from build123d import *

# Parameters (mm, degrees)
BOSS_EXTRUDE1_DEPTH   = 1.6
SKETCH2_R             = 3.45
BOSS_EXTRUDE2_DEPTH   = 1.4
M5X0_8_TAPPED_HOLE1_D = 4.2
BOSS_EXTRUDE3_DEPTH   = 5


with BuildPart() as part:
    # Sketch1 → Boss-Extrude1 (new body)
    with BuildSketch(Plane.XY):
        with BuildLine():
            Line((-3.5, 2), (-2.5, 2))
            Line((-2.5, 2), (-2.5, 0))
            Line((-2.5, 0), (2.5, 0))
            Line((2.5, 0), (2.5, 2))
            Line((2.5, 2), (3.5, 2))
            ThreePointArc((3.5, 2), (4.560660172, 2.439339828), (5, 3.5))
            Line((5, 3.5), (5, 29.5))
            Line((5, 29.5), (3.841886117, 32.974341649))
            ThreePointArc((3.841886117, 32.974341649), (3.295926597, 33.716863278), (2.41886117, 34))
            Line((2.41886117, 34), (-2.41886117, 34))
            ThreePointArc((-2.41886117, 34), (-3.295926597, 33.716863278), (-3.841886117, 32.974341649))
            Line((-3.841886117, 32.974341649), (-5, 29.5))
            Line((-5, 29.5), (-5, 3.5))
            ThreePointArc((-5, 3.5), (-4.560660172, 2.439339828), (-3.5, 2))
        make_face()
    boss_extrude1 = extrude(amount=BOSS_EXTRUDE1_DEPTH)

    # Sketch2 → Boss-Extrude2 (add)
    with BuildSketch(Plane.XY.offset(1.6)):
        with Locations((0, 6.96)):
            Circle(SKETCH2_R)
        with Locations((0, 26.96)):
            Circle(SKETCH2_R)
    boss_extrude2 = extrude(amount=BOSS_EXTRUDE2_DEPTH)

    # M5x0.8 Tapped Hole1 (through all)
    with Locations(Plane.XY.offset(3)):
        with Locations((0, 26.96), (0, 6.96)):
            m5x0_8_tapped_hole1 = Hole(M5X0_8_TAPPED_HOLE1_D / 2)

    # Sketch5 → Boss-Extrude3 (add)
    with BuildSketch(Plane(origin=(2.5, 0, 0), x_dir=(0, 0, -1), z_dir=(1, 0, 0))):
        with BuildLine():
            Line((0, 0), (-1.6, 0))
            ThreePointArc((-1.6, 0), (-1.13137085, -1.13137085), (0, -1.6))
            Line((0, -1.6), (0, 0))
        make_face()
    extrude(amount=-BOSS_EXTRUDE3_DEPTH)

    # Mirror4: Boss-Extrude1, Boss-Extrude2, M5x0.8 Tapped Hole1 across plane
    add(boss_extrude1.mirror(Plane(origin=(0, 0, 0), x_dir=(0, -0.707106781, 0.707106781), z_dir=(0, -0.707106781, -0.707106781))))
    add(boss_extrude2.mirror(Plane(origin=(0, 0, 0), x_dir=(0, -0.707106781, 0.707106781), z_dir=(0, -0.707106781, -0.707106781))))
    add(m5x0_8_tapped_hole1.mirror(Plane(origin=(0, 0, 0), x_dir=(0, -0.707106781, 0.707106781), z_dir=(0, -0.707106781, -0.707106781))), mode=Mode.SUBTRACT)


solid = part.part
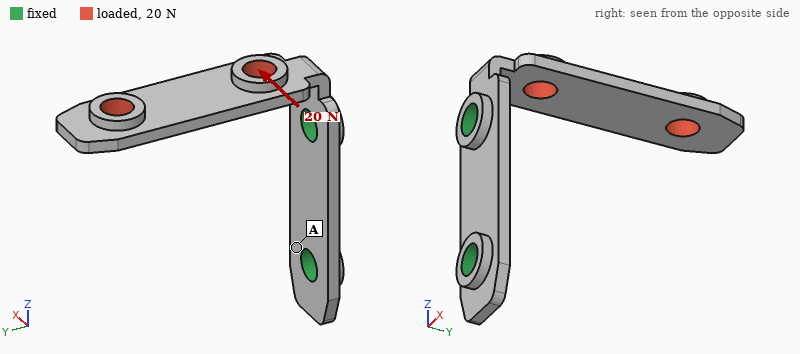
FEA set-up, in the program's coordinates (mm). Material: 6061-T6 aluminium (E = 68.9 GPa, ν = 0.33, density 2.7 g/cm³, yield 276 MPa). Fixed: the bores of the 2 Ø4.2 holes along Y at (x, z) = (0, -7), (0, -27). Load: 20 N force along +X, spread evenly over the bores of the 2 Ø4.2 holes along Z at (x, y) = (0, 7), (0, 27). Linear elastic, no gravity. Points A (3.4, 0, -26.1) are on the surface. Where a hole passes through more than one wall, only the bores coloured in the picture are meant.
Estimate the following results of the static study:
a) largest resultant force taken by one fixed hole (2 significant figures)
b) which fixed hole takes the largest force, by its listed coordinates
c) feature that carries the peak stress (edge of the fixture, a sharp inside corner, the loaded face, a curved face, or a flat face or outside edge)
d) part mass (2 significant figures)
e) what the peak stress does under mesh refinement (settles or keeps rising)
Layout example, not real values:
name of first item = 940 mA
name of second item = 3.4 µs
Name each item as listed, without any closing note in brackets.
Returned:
largest resultant force taken by one fixed hole = 21 N
which fixed hole takes the largest force, by its listed coordinates = (0, -7)
feature that carries the peak stress = a sharp inside corner
part mass = 2.9 g
what the peak stress does under mesh refinement = keeps rising
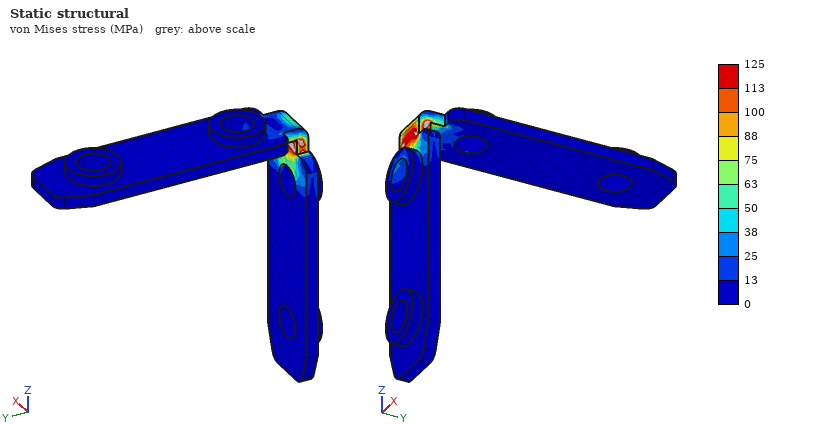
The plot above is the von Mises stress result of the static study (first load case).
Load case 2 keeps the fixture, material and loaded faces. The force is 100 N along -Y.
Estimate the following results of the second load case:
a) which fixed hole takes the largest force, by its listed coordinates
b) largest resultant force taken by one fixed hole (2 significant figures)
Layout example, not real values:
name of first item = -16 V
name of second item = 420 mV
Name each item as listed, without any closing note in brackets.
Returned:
which fixed hole takes the largest force, by its listed coordinates = (0, -7)
largest resultant force taken by one fixed hole = 100 N
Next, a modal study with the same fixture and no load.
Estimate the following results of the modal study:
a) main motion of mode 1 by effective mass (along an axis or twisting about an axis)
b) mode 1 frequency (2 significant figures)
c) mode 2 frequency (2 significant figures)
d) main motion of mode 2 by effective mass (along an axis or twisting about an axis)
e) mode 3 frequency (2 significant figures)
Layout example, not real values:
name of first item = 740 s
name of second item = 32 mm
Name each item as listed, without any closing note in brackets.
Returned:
main motion of mode 1 by effective mass = along Z
mode 1 frequency = 720 Hz
mode 2 frequency = 1300 Hz
main motion of mode 2 by effective mass = along X
mode 3 frequency = 5300 Hz
